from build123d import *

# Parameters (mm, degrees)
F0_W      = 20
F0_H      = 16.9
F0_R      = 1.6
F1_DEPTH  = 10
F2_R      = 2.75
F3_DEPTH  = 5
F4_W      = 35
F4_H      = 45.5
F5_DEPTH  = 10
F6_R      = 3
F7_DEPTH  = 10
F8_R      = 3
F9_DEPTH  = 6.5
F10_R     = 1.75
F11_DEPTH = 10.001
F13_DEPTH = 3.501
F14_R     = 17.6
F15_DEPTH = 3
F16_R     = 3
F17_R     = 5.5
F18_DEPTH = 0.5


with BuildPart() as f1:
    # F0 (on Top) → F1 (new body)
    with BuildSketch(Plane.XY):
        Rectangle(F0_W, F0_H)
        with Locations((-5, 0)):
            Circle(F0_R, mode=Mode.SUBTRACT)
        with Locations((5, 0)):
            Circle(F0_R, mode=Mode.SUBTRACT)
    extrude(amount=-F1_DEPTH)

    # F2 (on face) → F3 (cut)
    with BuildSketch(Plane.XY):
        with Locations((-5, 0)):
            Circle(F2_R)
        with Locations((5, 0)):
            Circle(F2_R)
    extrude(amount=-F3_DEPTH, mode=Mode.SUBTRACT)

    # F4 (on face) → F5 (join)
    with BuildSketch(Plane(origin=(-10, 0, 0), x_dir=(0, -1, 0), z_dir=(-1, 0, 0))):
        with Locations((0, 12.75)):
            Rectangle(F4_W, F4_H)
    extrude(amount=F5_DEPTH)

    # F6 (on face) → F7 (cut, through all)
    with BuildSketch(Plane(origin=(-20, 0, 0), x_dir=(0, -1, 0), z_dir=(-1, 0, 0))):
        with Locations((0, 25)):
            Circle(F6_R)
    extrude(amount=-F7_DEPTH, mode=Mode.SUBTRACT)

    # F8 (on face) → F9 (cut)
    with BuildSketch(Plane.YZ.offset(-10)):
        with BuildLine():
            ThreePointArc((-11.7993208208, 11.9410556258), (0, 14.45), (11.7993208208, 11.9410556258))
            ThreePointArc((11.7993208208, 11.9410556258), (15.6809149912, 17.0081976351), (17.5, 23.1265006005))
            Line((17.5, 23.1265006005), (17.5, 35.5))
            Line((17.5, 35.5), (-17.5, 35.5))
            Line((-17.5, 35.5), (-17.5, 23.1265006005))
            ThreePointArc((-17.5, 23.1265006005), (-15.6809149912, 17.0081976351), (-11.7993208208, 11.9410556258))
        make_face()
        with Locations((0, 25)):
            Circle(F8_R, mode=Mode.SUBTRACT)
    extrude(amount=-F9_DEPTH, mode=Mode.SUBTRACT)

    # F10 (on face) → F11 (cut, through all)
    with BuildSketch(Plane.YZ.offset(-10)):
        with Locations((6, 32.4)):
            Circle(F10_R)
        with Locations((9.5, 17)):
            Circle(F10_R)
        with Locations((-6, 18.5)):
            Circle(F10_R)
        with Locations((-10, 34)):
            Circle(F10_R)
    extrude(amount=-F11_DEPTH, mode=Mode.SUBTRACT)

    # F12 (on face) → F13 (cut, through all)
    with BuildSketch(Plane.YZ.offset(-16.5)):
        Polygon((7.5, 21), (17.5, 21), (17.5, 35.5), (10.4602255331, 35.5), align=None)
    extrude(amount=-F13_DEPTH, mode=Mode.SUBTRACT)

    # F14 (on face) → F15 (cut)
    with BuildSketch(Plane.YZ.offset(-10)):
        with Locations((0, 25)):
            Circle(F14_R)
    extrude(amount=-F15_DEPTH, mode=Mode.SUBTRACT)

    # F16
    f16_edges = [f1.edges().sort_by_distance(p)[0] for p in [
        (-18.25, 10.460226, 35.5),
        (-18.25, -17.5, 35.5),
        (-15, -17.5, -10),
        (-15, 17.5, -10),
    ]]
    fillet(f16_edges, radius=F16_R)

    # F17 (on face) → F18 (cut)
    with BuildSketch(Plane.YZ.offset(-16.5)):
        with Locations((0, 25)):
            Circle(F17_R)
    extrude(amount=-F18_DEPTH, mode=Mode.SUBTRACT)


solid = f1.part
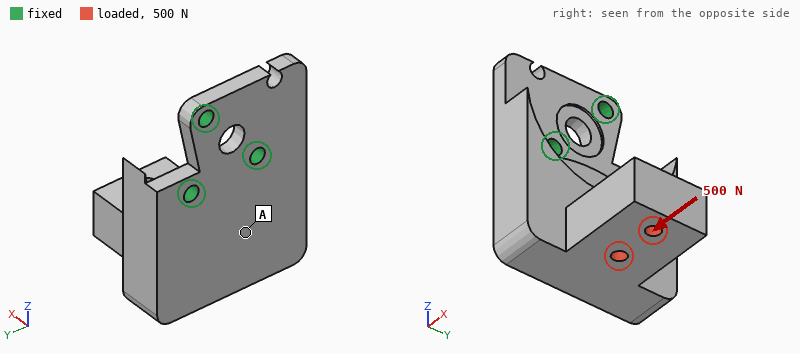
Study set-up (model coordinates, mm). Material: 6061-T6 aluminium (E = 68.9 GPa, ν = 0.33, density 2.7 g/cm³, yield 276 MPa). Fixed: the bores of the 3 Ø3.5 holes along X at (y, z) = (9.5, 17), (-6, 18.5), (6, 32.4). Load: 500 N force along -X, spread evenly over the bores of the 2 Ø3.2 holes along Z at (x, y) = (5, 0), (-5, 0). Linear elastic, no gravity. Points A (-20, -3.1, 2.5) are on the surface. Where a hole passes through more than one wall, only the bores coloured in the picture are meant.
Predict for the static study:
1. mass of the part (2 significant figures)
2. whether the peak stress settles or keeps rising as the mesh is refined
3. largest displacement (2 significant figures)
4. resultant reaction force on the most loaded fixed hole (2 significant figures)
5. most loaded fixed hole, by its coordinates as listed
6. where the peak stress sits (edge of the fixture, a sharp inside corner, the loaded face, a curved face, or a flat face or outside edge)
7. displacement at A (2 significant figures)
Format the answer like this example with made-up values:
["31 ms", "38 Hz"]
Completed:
["35 g", "keeps rising", "0.26 mm", "330 N", "(9.5, 17)", "edge of the fixture", "0.086 mm"]
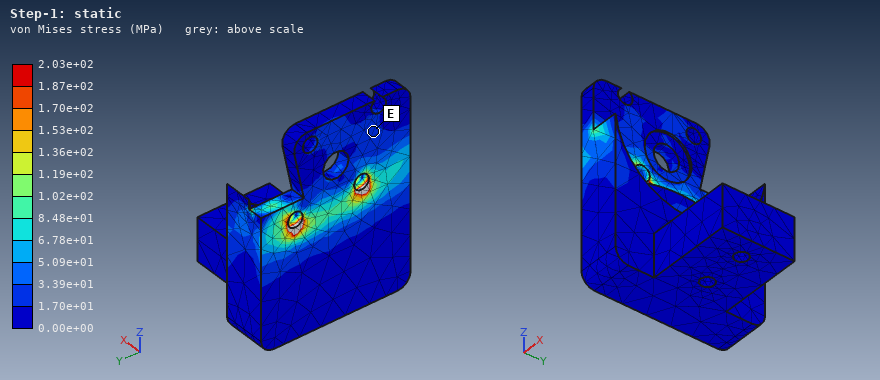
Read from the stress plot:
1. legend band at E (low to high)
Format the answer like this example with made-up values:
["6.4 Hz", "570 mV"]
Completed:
["1.70e+01 to 3.39e+01 MPa"]
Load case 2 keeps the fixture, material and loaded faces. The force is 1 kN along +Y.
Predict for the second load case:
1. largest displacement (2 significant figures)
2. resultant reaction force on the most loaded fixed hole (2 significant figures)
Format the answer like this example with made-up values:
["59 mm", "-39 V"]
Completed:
["94 µm", "1.7 kN"]
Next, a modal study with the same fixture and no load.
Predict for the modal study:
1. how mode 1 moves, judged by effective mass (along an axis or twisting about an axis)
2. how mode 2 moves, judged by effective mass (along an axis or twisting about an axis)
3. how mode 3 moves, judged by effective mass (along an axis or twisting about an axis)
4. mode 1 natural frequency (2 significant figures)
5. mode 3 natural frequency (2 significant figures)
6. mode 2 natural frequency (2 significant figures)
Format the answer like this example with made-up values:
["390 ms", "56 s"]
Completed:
["along X", "along Y", "along Y", "1900 Hz", "9700 Hz", "5700 Hz"]
